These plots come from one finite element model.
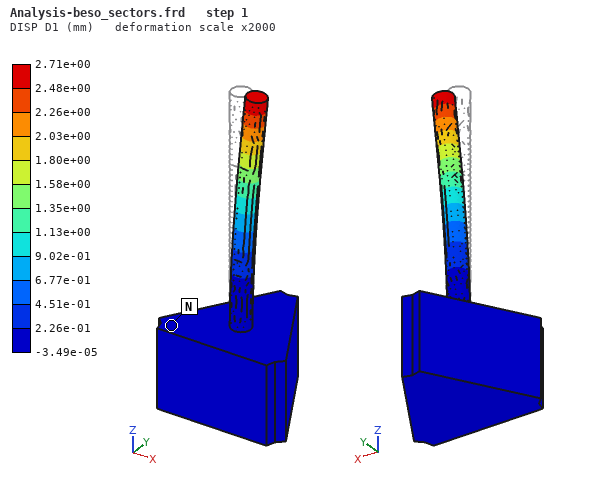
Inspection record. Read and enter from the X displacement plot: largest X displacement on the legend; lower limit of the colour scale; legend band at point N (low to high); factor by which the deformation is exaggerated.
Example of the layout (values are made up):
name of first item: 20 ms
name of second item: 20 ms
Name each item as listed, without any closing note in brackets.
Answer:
largest X displacement on the legend: 2.71e+00 mm
lower limit of the colour scale: -3.49e-05 mm
legend band at point N: -3.49e-05 to 2.26e-01 mm
factor by which the deformation is exaggerated: 2000
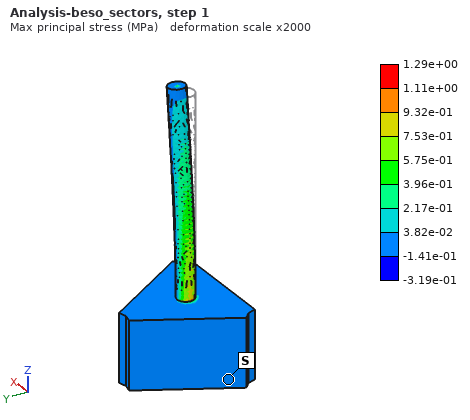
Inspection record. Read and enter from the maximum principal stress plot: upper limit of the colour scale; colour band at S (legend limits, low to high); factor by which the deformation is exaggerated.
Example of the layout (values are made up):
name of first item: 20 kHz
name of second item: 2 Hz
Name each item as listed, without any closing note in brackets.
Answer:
upper limit of the colour scale: 1.29e+00 MPa
colour band at S: -1.41e-01 to 3.82e-02 MPa
factor by which the deformation is exaggerated: 2000
